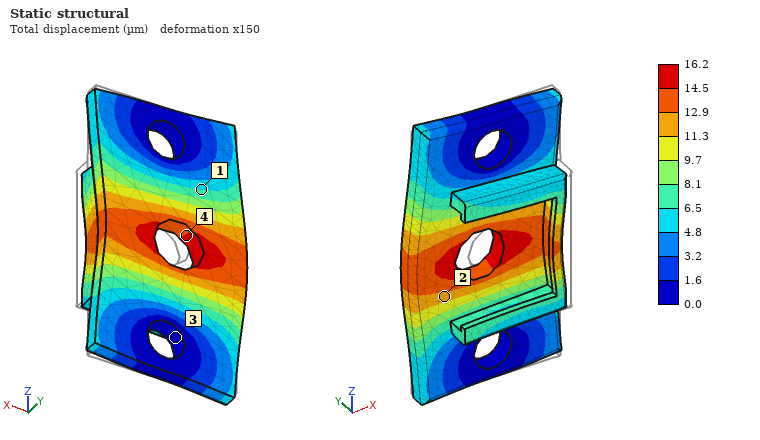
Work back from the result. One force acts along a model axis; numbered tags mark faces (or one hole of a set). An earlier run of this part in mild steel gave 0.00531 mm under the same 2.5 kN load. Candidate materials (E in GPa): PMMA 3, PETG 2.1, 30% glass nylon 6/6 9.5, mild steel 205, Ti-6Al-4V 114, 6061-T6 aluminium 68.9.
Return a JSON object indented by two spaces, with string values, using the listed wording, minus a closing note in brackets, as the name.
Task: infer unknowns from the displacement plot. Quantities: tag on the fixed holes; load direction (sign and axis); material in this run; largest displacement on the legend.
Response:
{
  "tag on the fixed holes": "3",
  "load direction": "-X",
  "material in this run": "6061-T6 aluminium",
  "largest displacement on the legend": "16.2 µm"
}
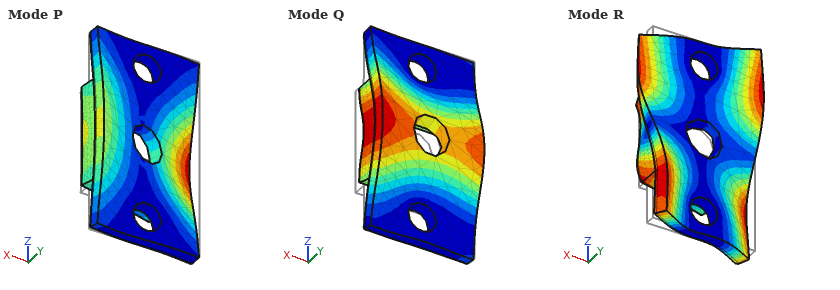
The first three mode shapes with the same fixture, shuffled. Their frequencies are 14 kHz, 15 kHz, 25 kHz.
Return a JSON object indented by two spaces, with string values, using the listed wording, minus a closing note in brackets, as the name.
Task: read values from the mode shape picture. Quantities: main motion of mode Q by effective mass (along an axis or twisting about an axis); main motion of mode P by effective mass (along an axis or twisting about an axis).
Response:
{
  "main motion of mode Q by effective mass": "along Y",
  "main motion of mode P by effective mass": "twisting about Z"
}
